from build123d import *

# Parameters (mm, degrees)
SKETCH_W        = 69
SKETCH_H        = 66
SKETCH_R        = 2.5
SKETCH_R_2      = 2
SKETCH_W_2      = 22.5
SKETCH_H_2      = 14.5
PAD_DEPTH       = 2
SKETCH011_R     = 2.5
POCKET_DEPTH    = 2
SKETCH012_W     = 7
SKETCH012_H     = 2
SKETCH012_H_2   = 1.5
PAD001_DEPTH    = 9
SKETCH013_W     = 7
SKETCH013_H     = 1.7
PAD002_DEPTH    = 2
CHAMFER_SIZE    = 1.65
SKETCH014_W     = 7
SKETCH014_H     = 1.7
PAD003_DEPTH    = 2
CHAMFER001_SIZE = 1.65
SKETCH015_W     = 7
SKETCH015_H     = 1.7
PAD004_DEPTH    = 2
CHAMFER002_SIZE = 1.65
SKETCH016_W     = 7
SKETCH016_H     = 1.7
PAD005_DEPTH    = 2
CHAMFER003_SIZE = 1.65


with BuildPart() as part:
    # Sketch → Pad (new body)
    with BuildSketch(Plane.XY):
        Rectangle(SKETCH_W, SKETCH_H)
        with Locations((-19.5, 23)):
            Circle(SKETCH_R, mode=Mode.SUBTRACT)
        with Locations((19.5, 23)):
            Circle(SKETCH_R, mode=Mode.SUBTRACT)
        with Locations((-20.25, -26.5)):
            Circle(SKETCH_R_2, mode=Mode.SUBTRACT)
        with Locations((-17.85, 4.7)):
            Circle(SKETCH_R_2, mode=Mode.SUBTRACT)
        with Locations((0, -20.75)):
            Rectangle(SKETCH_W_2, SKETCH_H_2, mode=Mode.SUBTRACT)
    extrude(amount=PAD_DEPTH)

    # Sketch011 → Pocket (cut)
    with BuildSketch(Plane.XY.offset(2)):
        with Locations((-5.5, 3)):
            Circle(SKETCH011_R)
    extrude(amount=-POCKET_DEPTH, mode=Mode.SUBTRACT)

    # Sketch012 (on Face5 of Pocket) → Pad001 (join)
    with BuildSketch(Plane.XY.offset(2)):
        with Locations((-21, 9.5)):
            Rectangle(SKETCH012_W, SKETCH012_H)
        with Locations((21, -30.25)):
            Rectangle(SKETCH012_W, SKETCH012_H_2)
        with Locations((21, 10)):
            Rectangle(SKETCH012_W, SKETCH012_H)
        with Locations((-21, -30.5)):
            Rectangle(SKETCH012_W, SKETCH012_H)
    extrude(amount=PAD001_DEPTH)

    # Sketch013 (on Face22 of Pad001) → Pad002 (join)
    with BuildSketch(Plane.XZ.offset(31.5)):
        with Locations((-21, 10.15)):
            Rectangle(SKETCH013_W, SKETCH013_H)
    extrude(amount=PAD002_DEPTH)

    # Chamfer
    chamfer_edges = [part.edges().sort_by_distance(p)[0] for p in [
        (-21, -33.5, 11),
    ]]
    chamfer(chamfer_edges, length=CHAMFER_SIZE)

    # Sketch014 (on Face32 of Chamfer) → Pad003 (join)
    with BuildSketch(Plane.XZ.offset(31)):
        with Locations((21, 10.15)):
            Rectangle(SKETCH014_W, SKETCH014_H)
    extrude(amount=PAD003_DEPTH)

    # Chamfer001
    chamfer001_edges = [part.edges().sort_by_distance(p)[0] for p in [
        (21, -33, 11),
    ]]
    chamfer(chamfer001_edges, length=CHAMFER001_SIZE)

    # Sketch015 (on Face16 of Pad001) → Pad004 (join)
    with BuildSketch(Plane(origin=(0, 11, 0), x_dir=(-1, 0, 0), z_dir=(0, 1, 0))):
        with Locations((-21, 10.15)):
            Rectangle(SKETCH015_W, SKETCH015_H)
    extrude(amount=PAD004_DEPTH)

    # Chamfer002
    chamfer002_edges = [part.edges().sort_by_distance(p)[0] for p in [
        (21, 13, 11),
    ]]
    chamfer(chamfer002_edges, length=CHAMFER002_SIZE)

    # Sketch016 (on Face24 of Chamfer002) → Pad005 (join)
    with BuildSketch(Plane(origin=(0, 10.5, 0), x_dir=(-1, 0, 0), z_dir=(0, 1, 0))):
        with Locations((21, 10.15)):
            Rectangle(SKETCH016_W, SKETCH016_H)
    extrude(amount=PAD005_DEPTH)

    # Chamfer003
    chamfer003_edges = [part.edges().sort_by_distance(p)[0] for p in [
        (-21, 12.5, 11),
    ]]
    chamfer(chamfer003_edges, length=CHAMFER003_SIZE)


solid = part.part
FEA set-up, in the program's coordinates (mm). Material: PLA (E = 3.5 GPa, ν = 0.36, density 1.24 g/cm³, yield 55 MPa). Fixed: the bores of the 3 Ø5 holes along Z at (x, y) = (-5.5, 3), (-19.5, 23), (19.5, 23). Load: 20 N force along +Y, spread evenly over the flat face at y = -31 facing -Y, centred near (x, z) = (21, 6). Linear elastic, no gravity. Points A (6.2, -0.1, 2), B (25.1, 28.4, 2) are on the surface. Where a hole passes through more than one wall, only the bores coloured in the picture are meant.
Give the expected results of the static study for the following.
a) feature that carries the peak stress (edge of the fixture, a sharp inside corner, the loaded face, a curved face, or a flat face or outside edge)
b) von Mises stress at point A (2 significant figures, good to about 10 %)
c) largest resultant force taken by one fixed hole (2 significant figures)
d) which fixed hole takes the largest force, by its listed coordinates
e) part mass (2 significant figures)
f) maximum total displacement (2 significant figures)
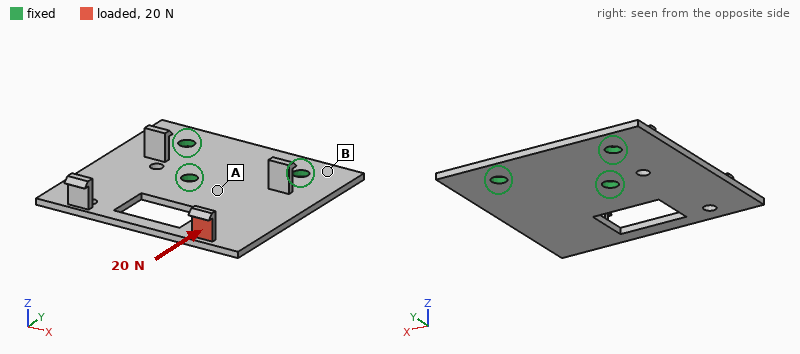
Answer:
the loaded face
2.2 MPa
17 N
(19.5, 23)
11 g
1.1 mm
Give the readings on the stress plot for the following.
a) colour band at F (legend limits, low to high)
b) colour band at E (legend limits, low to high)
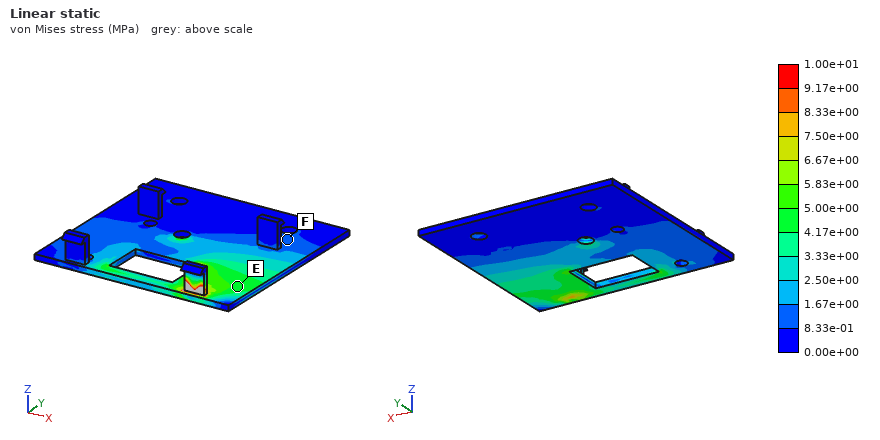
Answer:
8.33e-01 to 1.67e+00 MPa
4.17e+00 to 5.00e+00 MPa
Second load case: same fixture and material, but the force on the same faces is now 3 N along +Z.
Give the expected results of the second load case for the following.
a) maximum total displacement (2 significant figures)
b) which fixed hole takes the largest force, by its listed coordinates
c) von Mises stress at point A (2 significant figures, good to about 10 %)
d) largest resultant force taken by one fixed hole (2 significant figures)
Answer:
0.94 mm
(-5.5, 3)
2.6 MPa
4.1 N
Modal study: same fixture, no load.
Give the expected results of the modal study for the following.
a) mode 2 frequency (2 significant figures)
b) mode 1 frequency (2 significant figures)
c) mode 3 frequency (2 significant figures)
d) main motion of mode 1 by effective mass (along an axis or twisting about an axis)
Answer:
370 Hz
300 Hz
880 Hz
along Z
